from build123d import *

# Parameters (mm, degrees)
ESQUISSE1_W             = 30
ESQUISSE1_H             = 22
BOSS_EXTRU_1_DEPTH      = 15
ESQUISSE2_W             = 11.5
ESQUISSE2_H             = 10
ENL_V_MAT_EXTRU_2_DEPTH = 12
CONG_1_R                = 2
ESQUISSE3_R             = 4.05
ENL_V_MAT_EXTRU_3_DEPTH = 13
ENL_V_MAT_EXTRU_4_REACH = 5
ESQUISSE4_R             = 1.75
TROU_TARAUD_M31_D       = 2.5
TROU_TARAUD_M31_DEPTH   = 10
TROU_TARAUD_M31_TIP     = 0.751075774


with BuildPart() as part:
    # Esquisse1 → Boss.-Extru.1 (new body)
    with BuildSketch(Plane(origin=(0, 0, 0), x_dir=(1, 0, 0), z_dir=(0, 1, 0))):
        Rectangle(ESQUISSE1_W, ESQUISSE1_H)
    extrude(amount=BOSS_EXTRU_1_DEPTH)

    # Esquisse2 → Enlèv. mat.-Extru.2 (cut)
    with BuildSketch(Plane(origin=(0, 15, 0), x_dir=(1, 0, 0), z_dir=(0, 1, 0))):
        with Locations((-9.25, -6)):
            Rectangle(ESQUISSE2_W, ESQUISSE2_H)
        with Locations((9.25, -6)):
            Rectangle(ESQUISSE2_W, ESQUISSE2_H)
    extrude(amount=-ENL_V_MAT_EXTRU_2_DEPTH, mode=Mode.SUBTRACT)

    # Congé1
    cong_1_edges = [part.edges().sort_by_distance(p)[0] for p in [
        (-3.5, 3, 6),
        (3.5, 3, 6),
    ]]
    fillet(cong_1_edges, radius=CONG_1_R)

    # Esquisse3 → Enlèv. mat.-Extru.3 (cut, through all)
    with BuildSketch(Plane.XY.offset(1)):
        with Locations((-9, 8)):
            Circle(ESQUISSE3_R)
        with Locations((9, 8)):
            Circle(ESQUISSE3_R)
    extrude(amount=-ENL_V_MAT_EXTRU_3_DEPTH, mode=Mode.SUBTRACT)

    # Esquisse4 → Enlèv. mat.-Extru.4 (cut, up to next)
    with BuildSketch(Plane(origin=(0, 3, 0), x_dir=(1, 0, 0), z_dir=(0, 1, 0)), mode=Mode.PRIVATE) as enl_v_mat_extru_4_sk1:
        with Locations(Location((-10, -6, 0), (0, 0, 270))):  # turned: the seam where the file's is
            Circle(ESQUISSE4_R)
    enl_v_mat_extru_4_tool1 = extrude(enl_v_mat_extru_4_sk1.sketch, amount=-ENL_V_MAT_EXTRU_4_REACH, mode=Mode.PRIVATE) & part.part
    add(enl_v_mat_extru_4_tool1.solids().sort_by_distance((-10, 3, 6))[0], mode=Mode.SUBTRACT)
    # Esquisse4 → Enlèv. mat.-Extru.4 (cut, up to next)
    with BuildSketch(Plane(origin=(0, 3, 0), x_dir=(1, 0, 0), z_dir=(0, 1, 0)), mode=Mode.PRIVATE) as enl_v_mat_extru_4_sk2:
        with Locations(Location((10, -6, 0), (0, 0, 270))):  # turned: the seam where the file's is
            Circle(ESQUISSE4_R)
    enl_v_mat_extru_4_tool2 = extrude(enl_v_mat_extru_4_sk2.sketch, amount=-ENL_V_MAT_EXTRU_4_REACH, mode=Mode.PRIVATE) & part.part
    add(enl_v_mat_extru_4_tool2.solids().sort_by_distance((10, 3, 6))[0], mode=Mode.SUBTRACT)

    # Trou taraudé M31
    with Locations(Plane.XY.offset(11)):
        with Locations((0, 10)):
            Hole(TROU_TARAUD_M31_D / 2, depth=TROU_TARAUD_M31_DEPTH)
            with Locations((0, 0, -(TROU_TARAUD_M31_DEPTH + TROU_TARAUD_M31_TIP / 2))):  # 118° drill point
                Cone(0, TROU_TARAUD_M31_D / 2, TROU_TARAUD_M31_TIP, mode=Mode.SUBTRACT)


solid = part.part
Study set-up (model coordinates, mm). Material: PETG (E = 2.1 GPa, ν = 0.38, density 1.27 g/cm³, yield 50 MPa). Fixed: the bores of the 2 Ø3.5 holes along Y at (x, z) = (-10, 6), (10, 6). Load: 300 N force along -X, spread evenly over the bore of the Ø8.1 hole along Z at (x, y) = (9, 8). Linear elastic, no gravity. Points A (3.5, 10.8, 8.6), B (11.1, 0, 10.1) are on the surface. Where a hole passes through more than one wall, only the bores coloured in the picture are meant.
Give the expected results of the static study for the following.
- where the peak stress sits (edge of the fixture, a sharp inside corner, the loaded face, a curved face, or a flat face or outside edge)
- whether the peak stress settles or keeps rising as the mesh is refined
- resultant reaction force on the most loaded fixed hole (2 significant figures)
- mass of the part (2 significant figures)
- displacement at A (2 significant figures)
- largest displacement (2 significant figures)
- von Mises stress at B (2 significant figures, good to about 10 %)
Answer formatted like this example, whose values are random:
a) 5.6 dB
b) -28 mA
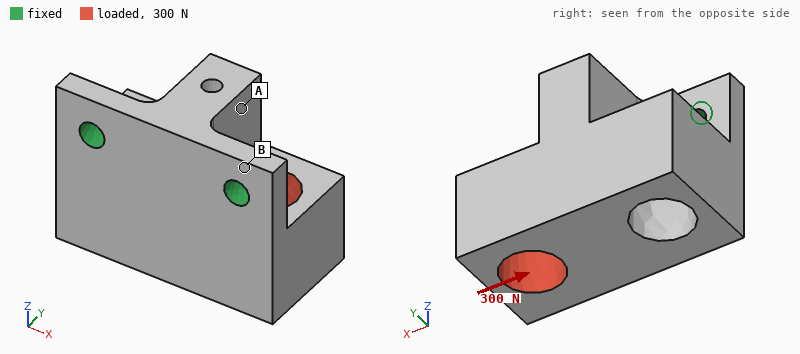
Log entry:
a) edge of the fixture
b) keeps rising
c) 240 N
d) 7.4 g
e) 0.061 mm
f) 0.15 mm
g) 4.0 MPa
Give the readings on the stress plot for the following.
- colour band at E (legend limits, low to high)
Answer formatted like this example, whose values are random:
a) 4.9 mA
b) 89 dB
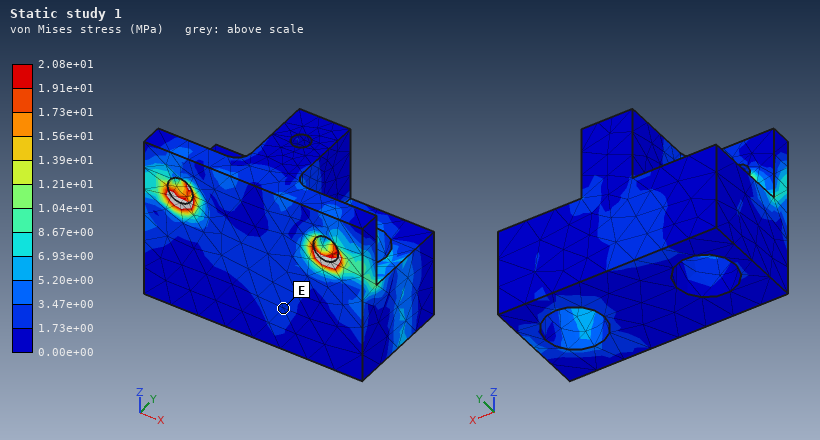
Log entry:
a) 1.73e+00 to 3.47e+00 MPa
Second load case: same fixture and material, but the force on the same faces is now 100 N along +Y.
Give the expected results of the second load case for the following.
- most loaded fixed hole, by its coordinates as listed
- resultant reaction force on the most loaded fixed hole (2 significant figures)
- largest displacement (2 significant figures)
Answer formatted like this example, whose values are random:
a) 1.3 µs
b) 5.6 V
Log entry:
a) (10, 6)
b) 95 N
c) 0.45 mm
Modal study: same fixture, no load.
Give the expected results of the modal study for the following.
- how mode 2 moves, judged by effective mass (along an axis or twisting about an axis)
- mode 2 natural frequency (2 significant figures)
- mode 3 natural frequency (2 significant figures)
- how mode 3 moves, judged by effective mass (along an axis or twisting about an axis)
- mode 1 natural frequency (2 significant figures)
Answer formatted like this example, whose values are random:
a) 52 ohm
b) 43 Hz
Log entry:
a) along X
b) 3100 Hz
c) 5000 Hz
d) along X
e) 1100 Hz
